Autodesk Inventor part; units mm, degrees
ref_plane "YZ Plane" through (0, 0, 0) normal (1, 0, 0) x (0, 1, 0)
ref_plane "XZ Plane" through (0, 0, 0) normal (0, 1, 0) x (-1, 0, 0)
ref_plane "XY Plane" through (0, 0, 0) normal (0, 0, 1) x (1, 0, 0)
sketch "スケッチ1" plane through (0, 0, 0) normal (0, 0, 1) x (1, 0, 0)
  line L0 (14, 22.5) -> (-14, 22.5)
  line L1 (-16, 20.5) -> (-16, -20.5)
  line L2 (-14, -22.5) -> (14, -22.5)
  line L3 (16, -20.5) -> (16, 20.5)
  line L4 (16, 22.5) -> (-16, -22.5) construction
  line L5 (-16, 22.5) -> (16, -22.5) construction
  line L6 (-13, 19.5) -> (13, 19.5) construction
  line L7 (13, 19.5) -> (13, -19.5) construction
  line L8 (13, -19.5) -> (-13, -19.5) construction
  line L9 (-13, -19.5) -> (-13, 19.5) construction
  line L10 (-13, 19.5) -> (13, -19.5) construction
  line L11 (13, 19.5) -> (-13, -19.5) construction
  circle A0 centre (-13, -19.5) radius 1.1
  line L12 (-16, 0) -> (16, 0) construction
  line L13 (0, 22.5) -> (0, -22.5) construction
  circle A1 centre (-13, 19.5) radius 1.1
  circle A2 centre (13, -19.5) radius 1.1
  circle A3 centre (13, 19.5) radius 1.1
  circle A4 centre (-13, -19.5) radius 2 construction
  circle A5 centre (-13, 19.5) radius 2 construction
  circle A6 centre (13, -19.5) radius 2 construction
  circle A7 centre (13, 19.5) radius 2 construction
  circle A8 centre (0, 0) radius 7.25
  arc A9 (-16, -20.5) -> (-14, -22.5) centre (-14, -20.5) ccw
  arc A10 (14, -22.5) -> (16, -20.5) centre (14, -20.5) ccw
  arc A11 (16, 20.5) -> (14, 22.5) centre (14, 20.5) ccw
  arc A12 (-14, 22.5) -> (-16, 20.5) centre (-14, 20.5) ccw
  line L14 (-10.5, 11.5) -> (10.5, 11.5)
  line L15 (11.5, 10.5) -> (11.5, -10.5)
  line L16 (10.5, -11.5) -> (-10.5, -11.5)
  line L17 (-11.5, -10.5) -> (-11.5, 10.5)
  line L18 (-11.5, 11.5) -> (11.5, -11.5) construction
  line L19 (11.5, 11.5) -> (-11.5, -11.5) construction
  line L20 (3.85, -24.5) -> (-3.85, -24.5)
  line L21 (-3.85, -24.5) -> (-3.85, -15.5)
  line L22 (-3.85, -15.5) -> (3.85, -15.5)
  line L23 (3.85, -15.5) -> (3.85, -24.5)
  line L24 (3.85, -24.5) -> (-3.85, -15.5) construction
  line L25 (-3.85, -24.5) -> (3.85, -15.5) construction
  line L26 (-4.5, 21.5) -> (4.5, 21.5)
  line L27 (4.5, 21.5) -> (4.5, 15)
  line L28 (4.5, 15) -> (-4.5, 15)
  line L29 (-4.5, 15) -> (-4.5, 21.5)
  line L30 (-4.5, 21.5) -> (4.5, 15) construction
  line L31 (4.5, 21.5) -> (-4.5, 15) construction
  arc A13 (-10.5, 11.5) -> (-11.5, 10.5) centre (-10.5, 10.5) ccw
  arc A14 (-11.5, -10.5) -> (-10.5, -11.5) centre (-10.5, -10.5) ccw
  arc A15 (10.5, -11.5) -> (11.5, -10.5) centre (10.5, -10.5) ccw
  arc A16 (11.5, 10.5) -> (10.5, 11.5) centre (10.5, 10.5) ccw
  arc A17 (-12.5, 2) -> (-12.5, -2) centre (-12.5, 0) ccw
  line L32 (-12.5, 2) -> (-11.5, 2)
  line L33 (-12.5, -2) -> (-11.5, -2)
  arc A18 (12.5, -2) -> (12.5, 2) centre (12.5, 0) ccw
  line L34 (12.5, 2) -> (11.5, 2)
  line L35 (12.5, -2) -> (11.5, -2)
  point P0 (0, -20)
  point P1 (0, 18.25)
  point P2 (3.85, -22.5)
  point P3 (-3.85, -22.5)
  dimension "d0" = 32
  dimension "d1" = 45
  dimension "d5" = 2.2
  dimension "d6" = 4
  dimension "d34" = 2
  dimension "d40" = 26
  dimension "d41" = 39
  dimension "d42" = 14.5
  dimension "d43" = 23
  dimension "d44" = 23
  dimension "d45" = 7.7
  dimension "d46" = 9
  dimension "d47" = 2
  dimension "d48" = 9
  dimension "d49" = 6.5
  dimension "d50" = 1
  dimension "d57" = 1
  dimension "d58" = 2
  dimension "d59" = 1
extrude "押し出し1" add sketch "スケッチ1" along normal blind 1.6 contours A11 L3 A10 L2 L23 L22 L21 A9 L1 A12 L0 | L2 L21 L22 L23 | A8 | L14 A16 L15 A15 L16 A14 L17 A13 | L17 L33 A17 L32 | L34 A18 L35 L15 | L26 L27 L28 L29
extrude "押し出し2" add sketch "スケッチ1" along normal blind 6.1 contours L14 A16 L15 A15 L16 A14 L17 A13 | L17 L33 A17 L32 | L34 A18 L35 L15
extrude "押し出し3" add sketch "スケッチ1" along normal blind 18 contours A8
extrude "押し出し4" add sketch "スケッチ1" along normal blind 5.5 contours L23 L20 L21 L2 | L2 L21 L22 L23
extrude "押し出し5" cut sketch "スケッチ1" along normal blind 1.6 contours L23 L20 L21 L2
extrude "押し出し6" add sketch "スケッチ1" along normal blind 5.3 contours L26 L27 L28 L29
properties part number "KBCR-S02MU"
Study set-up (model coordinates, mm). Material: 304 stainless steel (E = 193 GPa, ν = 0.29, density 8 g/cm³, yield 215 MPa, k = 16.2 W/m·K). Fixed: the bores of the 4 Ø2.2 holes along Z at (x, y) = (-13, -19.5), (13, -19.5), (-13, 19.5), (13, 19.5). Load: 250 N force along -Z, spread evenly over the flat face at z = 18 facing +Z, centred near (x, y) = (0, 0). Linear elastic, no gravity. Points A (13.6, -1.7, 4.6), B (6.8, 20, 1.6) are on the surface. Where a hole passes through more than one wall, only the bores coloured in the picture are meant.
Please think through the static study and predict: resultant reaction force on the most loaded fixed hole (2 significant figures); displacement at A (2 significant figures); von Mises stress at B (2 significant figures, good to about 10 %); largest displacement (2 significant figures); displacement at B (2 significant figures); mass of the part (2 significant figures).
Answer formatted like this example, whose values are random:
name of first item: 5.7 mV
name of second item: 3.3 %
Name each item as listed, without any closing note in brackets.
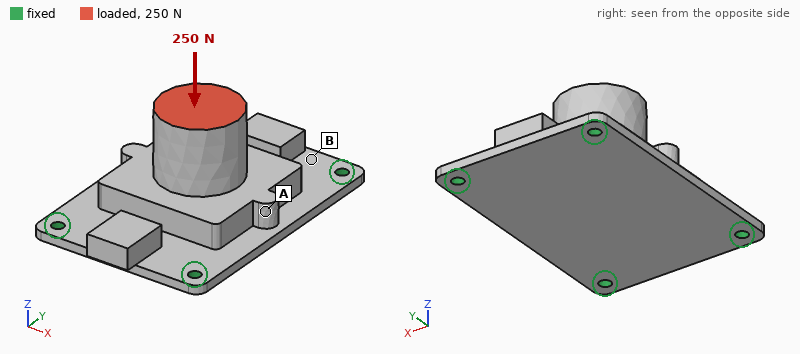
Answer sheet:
resultant reaction force on the most loaded fixed hole: 79 N
displacement at A: 7.6 µm
von Mises stress at B: 13 MPa
largest displacement: 7.8 µm
displacement at B: 1.4 µm
mass of the part: 58 g
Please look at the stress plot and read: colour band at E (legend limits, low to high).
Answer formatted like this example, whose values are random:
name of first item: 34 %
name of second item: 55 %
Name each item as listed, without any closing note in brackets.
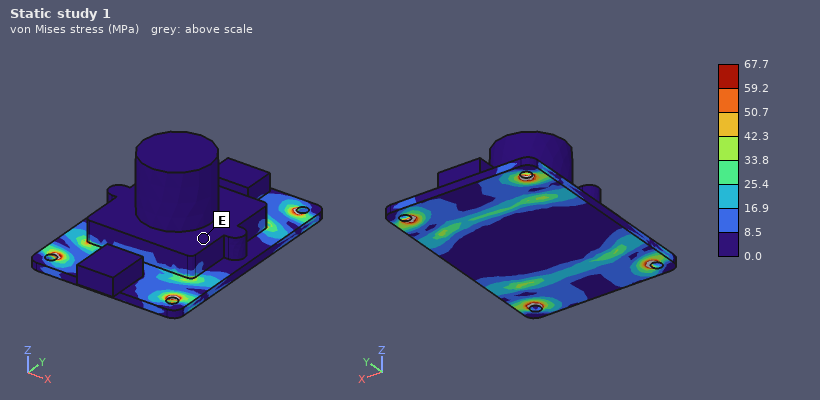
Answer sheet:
colour band at E: 0.0 to 8.5 MPa
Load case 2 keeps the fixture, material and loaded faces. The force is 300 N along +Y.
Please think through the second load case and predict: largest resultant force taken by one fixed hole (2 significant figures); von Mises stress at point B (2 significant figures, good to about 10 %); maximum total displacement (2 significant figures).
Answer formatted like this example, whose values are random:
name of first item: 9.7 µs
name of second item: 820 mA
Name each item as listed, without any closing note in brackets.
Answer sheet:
largest resultant force taken by one fixed hole: 120 N
von Mises stress at point B: 14 MPa
maximum total displacement: 13 µm
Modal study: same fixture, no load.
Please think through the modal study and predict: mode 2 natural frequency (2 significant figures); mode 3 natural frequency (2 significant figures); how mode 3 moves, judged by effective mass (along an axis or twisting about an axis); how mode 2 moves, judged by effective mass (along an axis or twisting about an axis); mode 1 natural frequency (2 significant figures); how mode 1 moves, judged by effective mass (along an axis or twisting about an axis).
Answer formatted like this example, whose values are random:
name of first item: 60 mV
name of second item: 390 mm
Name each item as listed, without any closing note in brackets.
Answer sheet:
mode 2 natural frequency: 5200 Hz
mode 3 natural frequency: 6900 Hz
how mode 3 moves, judged by effective mass: along Y
how mode 2 moves, judged by effective mass: along X
mode 1 natural frequency: 4200 Hz
how mode 1 moves, judged by effective mass: along Z
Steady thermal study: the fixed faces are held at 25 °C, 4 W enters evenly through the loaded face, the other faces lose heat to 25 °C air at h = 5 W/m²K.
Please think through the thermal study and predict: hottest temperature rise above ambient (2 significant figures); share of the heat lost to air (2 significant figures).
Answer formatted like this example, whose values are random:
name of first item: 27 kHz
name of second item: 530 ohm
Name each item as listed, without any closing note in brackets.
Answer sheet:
hottest temperature rise above ambient: 56 K
share of the heat lost to air: 14 %
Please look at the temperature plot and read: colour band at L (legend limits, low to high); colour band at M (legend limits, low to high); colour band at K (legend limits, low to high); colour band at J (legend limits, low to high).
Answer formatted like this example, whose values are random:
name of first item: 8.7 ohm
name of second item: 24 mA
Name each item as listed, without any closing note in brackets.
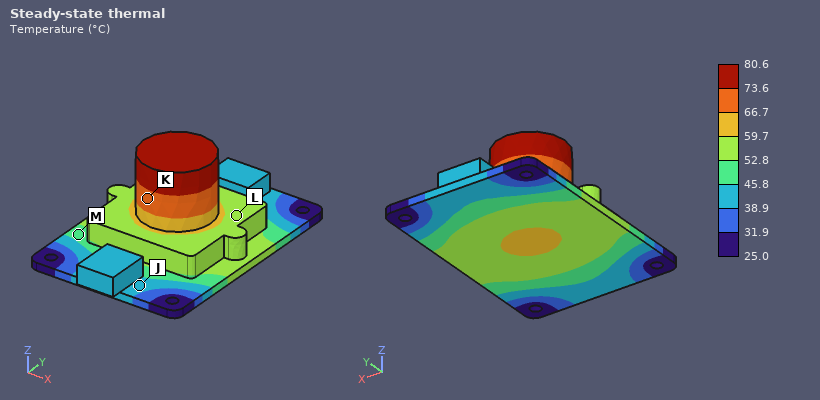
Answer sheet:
colour band at L: 52.8 to 59.7 °C
colour band at M: 45.8 to 52.8 °C
colour band at K: 66.7 to 73.6 °C
colour band at J: 38.9 to 45.8 °C
